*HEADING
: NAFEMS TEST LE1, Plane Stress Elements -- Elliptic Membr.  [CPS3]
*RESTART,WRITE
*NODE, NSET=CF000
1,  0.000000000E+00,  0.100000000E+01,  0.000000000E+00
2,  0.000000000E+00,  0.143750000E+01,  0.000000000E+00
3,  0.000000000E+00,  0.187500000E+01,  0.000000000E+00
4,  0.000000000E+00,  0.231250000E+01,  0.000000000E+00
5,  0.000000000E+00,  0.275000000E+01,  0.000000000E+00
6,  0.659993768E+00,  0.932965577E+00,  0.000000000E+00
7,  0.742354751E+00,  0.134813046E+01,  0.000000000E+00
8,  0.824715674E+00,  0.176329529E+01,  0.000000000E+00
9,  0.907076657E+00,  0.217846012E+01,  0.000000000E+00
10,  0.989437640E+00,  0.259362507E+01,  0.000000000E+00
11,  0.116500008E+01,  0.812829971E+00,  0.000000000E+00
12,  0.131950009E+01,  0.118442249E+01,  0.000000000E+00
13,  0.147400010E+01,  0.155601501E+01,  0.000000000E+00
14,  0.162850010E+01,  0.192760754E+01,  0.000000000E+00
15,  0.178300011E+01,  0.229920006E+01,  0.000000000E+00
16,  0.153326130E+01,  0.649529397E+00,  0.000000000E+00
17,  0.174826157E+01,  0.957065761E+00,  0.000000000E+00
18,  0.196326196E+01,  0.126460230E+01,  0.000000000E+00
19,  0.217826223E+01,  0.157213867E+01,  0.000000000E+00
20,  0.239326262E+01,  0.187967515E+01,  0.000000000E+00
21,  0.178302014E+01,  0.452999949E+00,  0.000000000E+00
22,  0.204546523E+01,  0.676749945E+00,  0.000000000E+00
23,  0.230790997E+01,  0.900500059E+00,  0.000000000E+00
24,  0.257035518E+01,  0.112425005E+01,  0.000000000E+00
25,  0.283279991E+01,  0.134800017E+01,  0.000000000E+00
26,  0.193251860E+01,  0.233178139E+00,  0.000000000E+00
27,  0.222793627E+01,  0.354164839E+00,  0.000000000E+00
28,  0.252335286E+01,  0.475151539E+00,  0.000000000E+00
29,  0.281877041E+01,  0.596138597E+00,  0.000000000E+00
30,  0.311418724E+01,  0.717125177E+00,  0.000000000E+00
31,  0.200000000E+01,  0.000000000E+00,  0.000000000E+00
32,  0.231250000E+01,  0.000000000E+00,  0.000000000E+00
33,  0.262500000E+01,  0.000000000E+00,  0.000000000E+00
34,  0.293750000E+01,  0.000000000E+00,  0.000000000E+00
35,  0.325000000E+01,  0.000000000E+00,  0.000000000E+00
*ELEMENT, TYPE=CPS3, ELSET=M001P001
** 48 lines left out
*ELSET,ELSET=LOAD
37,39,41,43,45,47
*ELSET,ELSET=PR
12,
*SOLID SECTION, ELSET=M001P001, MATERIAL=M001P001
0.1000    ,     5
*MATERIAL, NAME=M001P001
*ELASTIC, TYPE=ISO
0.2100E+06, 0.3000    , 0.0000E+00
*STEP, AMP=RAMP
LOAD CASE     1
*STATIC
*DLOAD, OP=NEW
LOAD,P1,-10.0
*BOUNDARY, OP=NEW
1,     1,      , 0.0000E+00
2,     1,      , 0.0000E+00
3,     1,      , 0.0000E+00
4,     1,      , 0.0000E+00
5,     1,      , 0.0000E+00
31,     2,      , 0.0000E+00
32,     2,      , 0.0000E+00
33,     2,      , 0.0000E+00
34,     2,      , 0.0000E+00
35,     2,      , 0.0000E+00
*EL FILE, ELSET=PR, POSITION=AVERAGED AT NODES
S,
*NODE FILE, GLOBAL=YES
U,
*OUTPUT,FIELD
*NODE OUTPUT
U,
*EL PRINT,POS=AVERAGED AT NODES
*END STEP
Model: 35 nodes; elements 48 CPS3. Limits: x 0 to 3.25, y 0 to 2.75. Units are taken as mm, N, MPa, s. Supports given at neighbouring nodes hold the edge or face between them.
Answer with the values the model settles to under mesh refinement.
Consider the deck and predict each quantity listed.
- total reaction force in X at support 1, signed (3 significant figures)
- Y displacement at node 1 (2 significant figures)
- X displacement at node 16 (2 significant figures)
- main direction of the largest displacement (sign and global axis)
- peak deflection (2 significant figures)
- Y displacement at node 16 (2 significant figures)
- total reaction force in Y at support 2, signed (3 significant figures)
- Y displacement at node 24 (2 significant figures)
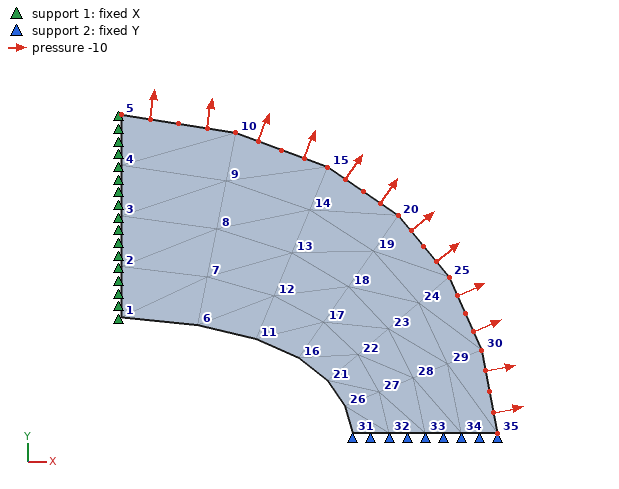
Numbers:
-2.75 N
5.5e-04 mm
-6.6e-05 mm
+Y
5.5e-04 mm
3.1e-04 mm
-3.25 N
9.0e-05 mm
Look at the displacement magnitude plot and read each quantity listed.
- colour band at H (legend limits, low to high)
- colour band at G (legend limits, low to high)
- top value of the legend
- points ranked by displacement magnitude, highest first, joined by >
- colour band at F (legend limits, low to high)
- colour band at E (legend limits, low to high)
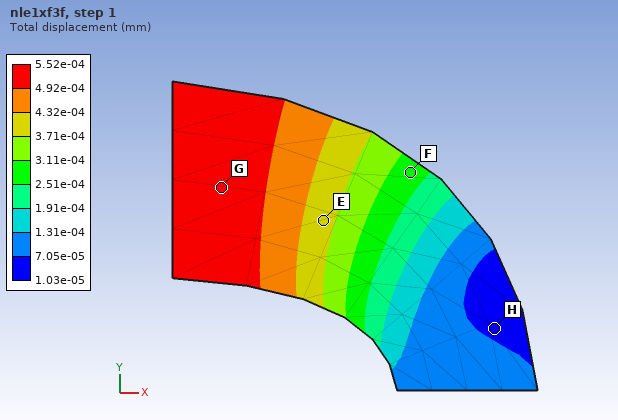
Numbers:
1.03e-05 to 7.05e-05 mm
4.92e-04 to 5.52e-04 mm
5.52e-04 mm
G > E > F > H
2.51e-04 to 3.11e-04 mm
3.71e-04 to 4.32e-04 mm
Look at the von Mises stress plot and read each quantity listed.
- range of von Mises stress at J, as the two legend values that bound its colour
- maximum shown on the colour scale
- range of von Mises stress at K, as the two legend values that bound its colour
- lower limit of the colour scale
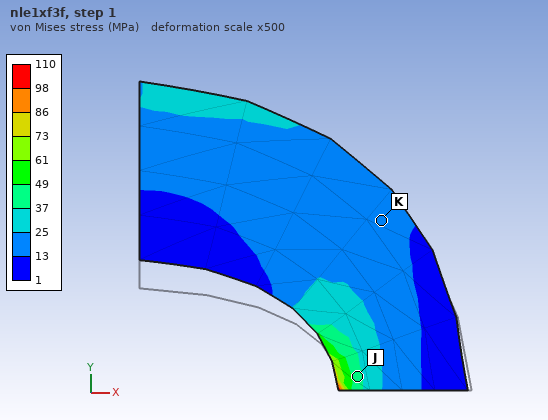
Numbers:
37 to 49 MPa
110 MPa
13 to 25 MPa
1 MPa
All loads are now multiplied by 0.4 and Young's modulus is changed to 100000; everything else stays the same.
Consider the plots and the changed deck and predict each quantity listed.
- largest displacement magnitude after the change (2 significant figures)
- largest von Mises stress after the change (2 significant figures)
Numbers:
4.6e-04 mm
44 MPa
